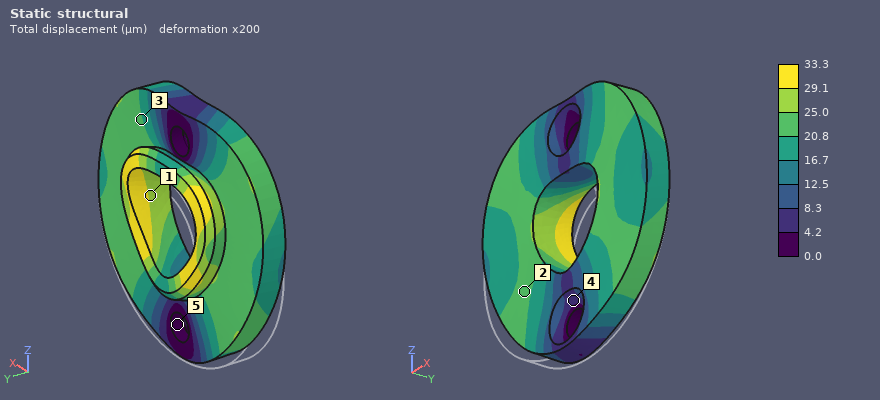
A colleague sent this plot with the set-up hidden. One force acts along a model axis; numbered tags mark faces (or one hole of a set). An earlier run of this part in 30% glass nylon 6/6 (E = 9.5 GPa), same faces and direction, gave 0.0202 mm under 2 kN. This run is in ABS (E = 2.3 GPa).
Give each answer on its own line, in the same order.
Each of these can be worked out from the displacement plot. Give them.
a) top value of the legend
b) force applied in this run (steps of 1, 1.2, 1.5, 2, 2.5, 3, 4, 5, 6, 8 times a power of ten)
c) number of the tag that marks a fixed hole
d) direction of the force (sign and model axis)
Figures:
33.3 µm
800 N
5
+Z
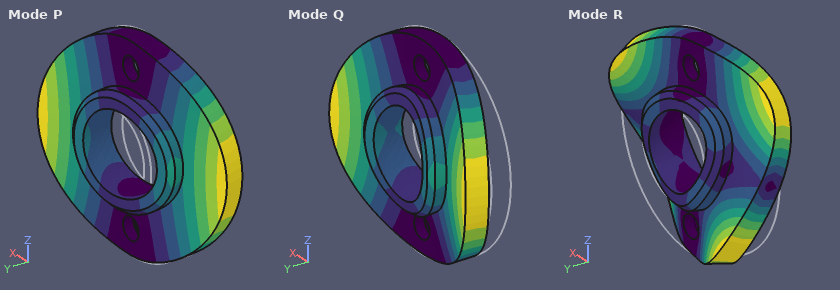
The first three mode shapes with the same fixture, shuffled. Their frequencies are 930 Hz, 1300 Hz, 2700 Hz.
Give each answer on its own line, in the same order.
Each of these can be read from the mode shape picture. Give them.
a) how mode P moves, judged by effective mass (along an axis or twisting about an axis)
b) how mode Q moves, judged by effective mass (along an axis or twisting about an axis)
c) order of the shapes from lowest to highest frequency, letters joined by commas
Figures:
twisting about Z
along Y
P, Q, R
